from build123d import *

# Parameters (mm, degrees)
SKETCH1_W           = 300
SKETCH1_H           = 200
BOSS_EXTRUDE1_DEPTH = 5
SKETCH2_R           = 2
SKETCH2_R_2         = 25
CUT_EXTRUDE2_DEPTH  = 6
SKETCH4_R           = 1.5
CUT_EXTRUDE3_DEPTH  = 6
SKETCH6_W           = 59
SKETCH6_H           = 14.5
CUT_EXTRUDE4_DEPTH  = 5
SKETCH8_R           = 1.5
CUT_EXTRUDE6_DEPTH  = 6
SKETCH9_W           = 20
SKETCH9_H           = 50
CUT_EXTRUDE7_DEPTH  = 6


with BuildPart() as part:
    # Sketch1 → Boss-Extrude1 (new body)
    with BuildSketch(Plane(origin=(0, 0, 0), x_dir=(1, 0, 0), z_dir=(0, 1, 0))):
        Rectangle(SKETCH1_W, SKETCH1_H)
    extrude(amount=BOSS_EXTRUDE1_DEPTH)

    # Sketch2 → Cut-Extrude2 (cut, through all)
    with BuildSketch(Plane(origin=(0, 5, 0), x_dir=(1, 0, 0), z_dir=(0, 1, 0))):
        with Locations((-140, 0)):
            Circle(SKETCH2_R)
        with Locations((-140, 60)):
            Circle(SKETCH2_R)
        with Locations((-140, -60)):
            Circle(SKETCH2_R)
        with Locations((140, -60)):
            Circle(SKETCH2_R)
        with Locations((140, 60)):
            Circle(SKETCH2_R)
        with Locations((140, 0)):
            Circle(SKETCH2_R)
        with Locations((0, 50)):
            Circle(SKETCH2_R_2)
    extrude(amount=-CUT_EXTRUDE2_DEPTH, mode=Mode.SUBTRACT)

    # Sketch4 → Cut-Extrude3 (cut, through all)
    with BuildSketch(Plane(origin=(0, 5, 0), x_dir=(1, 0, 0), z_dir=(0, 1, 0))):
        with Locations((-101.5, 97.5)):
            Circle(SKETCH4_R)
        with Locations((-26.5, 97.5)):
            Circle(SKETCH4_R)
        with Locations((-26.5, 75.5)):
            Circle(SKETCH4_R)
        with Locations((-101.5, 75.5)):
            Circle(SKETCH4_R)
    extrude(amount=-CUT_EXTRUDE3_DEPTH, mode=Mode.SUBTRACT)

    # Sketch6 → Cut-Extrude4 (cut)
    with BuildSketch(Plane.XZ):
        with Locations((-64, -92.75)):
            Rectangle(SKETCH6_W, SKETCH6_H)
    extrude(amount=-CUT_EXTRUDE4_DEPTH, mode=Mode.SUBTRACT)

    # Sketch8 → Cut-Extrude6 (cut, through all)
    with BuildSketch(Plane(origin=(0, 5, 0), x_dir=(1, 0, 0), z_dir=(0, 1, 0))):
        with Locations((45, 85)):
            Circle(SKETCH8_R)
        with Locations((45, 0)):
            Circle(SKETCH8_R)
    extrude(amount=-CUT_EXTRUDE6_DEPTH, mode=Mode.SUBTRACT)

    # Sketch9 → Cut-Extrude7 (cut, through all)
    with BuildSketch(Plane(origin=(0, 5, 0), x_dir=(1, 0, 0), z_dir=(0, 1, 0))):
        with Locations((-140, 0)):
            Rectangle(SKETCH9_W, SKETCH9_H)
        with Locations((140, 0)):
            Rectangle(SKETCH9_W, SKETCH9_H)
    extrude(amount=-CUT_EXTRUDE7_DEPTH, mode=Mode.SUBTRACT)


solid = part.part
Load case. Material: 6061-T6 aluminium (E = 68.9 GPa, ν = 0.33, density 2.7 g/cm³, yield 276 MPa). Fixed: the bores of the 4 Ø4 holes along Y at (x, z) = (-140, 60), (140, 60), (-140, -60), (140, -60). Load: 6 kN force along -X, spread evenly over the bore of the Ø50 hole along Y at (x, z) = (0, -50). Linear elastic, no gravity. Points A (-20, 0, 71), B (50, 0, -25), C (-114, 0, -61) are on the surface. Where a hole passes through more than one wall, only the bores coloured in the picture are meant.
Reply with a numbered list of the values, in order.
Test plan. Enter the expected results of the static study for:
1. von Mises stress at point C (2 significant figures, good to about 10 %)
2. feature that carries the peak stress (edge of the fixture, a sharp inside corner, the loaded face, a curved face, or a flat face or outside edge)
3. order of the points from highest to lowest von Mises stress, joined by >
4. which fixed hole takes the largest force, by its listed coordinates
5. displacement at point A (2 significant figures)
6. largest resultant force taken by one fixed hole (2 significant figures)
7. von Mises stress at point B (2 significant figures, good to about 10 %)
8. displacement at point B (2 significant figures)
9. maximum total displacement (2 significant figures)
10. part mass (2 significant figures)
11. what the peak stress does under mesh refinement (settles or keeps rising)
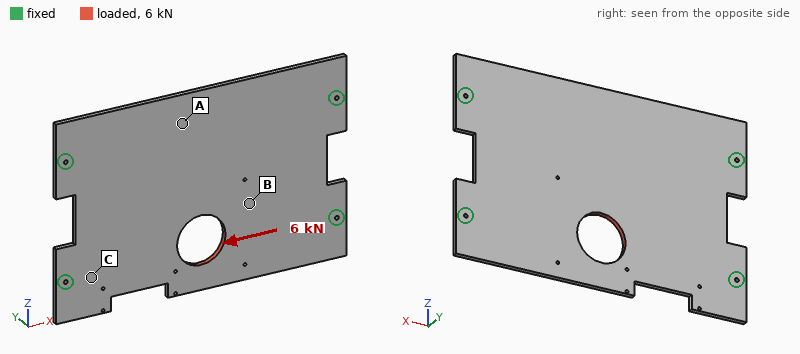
1. 10 MPa
2. edge of the fixture
3. C > B > A
4. (140, -60)
5. 4.7 µm
6. 2.1 kN
7. 5.2 MPa
8. 11 µm
9. 19 µm
10. 740 g
11. keeps rising
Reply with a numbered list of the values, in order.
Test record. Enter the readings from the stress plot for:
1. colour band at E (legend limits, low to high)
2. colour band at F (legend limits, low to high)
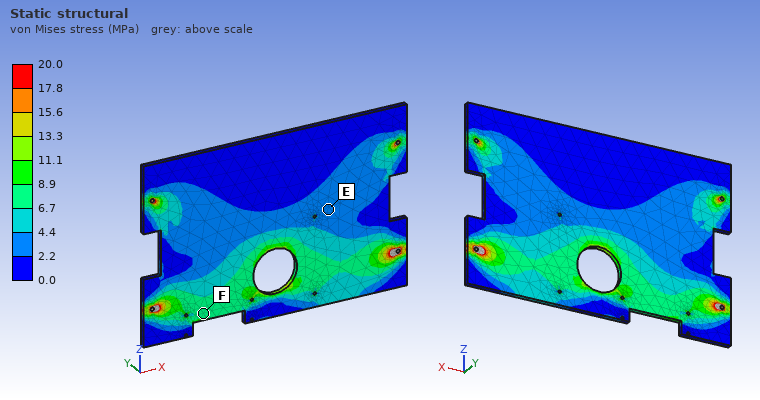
1. 2.2 to 4.4 MPa
2. 6.7 to 8.9 MPa
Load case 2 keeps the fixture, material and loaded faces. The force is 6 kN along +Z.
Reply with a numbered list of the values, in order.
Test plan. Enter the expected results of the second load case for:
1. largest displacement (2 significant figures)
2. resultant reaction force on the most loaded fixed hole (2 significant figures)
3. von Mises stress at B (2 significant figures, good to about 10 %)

1. 41 µm
2. 2.0 kN
3. 8.8 MPa
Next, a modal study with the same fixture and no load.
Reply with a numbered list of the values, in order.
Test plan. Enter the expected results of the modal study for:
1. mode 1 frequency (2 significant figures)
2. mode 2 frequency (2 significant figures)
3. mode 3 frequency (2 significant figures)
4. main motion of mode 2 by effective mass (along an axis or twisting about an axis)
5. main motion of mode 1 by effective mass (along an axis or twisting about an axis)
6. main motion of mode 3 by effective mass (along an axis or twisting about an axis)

1. 270 Hz
2. 400 Hz
3. 760 Hz
4. twisting about X
5. along Y
6. twisting about Z
